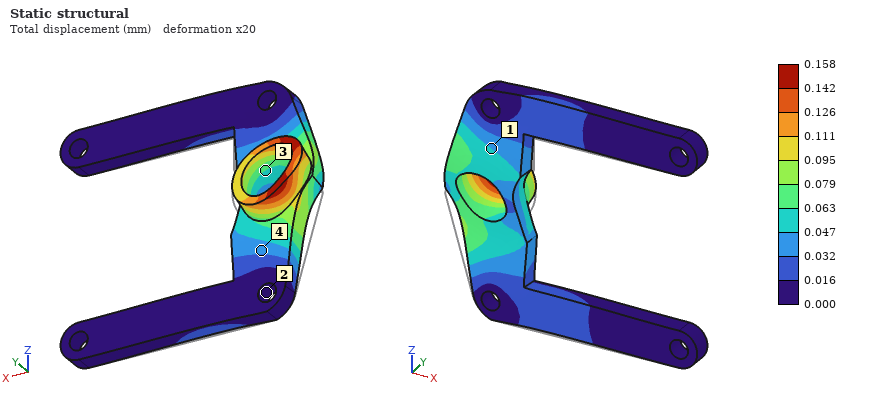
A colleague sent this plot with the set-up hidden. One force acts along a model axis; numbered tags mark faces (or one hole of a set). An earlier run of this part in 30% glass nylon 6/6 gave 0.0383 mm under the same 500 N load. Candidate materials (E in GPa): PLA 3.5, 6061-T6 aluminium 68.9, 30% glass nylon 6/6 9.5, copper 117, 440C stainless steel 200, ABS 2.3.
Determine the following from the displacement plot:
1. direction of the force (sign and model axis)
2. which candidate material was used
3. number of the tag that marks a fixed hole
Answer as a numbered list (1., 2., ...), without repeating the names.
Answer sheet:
1. +Z
2. ABS
3. 2
